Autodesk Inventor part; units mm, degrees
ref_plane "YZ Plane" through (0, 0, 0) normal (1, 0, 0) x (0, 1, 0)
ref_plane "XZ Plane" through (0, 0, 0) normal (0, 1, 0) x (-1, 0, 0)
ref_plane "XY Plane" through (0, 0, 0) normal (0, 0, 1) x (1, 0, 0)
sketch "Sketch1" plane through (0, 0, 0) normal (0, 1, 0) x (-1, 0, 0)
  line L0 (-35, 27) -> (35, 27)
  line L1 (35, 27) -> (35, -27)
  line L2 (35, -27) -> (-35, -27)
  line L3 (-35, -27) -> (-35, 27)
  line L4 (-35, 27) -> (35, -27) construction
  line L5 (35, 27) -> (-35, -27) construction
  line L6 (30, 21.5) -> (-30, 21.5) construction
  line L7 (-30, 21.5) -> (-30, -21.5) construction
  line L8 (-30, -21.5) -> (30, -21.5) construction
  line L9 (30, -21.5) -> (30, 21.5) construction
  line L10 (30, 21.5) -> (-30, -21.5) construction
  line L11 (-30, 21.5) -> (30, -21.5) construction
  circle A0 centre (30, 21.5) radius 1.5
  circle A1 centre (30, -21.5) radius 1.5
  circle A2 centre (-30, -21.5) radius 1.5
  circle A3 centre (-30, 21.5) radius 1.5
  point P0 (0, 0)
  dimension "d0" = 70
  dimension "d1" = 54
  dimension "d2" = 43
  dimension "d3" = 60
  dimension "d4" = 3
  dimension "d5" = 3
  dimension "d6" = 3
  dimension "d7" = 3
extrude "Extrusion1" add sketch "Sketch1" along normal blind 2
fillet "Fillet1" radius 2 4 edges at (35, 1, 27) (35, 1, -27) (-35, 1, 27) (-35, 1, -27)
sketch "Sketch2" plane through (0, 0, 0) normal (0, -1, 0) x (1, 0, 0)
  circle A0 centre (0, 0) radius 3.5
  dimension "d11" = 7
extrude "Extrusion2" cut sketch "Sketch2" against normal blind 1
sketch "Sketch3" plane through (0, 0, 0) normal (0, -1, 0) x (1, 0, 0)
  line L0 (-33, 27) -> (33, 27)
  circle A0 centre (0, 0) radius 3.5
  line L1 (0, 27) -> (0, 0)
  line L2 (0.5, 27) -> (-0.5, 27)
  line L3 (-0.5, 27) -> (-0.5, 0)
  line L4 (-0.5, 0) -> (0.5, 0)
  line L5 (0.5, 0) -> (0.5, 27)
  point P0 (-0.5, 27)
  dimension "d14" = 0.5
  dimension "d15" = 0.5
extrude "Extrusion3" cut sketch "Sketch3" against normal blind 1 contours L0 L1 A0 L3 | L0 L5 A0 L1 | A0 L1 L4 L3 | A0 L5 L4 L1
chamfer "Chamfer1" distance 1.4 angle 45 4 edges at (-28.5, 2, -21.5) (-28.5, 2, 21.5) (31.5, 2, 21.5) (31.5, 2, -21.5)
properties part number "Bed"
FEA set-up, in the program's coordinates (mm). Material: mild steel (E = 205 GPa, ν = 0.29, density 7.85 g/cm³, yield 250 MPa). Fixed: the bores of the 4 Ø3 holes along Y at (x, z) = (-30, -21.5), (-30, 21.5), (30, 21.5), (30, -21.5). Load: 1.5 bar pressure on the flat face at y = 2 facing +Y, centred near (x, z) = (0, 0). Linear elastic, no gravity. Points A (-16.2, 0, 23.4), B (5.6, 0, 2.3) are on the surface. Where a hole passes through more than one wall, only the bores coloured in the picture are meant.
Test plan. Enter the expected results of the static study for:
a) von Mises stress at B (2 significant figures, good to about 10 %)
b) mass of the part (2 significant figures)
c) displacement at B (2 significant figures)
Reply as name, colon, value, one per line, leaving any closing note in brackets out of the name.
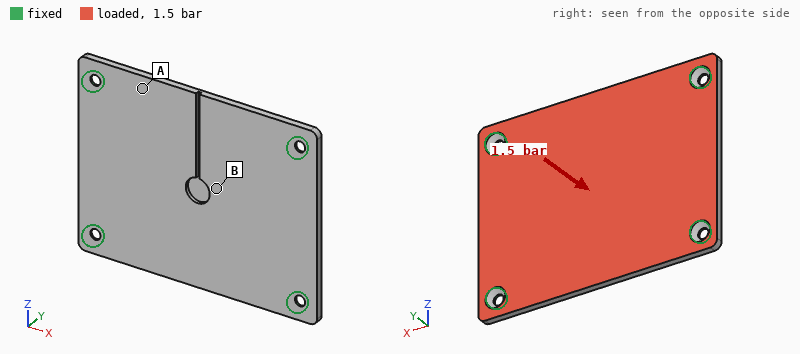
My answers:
von Mises stress at B: 28 MPa
mass of the part: 58 g
displacement at B: 83 µm
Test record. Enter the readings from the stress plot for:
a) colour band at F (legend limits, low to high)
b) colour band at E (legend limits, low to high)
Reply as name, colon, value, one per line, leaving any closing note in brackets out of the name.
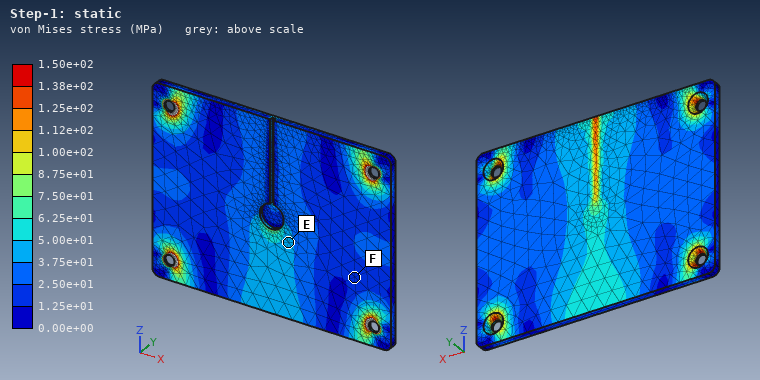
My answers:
colour band at F: 1.25e+01 to 2.50e+01 MPa
colour band at E: 3.75e+01 to 5.00e+01 MPa
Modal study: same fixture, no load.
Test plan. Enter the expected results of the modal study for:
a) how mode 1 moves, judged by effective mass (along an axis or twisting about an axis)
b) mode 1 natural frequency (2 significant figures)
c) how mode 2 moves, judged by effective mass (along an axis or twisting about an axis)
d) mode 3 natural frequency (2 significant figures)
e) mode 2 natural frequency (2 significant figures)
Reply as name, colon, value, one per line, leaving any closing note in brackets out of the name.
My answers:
how mode 1 moves, judged by effective mass: along Y
mode 1 natural frequency: 2000 Hz
how mode 2 moves, judged by effective mass: twisting about X
mode 3 natural frequency: 4500 Hz
mode 2 natural frequency: 3200 Hz
